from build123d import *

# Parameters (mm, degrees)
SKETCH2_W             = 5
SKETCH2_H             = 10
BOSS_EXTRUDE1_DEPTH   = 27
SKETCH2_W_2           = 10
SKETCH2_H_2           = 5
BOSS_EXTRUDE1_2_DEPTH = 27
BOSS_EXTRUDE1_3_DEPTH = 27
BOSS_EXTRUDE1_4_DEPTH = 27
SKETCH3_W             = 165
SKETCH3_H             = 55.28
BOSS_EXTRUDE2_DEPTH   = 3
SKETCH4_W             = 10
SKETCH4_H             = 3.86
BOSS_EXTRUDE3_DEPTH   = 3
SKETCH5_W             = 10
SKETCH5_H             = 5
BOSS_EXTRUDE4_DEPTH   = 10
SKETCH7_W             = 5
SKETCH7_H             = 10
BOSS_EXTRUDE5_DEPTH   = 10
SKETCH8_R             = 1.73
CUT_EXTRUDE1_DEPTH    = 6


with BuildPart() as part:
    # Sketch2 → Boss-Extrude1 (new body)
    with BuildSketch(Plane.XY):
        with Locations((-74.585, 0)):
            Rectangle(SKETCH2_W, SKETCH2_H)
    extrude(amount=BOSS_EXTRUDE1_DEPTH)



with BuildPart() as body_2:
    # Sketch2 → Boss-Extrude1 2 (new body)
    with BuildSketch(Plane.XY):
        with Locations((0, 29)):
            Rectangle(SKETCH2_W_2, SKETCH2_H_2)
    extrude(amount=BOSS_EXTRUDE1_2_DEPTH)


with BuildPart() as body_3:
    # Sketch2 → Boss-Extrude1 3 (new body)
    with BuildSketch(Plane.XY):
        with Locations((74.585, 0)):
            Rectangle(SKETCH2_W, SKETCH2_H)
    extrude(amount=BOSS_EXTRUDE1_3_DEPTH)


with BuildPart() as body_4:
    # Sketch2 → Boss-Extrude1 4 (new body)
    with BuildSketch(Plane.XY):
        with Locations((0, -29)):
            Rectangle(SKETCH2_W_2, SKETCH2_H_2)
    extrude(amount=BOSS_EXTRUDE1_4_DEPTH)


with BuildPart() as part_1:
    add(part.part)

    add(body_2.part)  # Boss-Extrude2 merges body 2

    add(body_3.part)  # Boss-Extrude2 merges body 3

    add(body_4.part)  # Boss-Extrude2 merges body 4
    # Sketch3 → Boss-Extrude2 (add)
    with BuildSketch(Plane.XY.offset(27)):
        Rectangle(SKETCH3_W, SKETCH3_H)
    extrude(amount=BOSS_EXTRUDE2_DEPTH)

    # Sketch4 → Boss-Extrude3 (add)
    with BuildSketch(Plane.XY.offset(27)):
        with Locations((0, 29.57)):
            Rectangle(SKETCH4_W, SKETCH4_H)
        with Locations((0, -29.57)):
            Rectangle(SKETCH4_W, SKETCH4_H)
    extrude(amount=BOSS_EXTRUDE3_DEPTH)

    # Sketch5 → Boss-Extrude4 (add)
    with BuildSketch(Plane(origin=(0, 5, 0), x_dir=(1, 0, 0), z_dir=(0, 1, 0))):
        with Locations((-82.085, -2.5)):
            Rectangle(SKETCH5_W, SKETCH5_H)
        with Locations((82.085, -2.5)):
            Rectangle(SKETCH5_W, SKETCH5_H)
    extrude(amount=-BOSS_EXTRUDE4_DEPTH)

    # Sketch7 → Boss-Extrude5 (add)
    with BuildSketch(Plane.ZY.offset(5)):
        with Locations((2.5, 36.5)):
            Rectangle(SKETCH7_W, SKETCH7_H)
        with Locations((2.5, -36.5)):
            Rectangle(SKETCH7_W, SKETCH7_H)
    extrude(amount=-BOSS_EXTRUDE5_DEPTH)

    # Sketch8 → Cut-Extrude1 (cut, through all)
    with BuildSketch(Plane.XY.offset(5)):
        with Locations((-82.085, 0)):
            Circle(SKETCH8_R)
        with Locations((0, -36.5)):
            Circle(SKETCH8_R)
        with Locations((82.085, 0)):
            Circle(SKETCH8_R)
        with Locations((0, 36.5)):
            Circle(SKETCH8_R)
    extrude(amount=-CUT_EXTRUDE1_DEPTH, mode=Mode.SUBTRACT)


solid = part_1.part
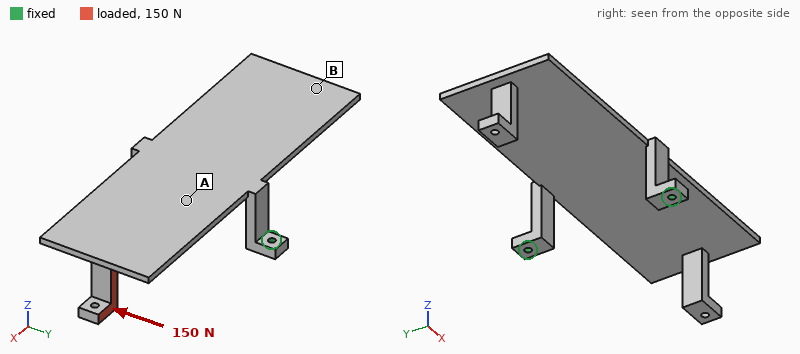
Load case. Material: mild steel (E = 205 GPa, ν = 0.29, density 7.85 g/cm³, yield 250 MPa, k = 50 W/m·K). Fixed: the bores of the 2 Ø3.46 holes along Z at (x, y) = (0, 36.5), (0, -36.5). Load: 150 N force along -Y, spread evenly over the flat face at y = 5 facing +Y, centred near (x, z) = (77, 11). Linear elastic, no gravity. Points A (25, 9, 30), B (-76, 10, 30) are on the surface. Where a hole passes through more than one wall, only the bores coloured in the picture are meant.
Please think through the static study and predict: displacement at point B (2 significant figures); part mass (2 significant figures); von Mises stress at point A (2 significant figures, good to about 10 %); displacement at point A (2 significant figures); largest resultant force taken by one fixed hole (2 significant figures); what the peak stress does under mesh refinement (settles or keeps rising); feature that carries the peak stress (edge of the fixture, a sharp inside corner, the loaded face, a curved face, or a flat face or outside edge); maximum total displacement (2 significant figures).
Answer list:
0.067 mm
270 g
25 MPa
0.050 mm
180 N
keeps rising
edge of the fixture
0.29 mm
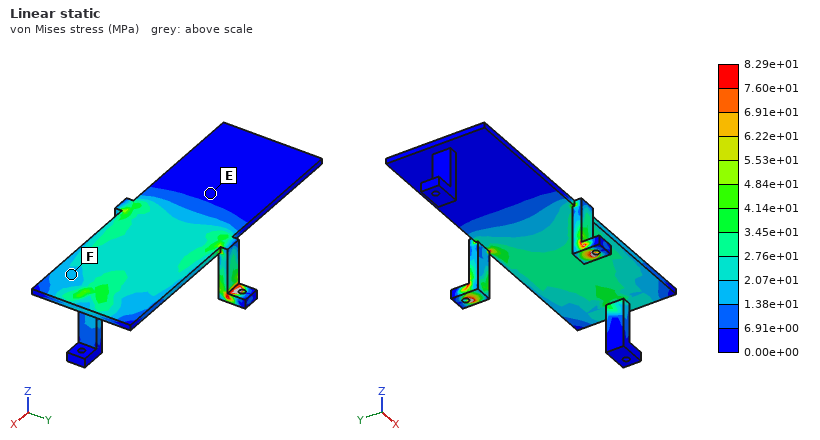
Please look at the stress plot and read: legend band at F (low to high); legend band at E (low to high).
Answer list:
1.38e+01 to 2.07e+01 MPa
0.00e+00 to 6.91e+00 MPa
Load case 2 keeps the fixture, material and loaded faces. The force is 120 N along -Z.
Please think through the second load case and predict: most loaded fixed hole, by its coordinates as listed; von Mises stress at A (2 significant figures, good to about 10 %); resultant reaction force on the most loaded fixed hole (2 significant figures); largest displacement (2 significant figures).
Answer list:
(0, 36.5)
78 MPa
85 N
1.3 mm
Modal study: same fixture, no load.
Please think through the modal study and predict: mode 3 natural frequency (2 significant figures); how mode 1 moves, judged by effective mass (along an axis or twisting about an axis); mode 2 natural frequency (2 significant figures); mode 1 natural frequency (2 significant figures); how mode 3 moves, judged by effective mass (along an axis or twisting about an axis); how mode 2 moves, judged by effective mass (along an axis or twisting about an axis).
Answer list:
590 Hz
twisting about Y
300 Hz
210 Hz
twisting about Z
along Z
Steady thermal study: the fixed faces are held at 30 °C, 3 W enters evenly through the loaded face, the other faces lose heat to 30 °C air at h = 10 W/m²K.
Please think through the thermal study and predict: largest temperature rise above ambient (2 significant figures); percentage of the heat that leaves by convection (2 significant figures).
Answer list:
45 K
74 %
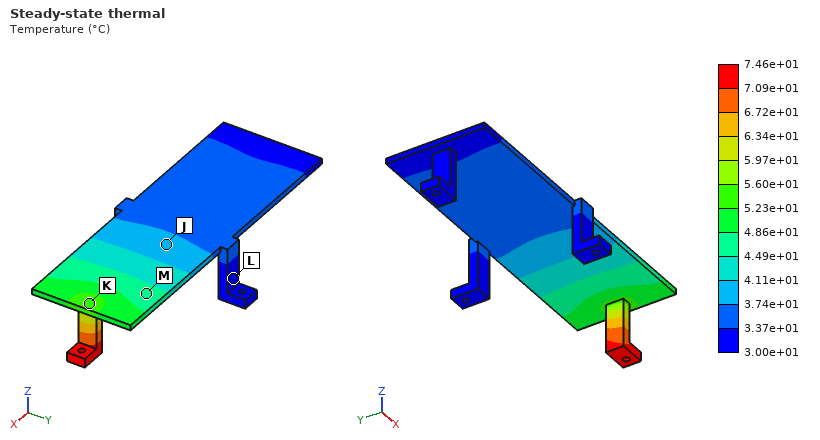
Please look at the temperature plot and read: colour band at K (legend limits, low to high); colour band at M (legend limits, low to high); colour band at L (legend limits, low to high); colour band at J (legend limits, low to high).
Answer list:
5.23e+01 to 5.60e+01 °C
4.49e+01 to 4.86e+01 °C
3.00e+01 to 3.37e+01 °C
3.74e+01 to 4.11e+01 °C
